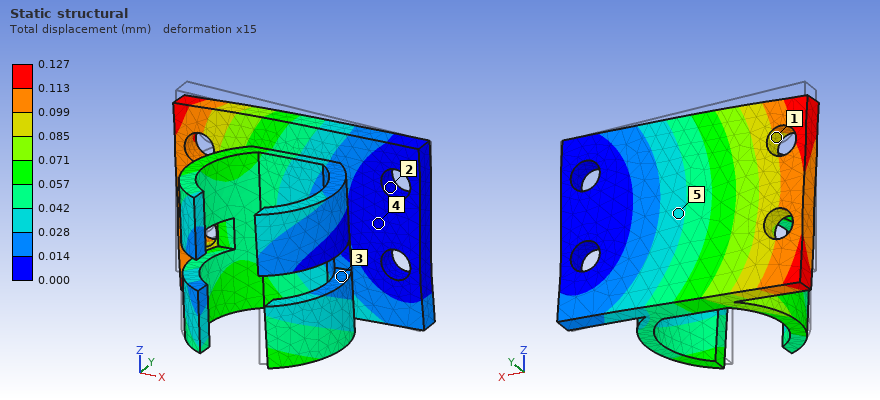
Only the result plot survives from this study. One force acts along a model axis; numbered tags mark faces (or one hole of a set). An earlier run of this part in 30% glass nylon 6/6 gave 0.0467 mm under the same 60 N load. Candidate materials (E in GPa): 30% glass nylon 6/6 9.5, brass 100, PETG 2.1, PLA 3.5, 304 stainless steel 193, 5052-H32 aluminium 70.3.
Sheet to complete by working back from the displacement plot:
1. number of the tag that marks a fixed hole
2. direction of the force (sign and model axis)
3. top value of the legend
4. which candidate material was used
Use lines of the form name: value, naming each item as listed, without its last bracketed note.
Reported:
number of the tag that marks a fixed hole: 2
direction of the force: -Z
top value of the legend: 0.127 mm
which candidate material was used: PLA
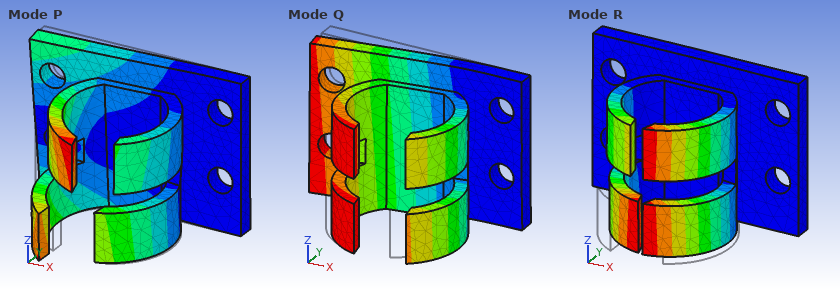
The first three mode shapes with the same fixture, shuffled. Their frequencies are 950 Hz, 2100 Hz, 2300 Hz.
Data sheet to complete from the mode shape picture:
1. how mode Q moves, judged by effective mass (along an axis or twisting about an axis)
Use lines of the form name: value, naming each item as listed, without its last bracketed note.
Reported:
how mode Q moves, judged by effective mass: along Y
